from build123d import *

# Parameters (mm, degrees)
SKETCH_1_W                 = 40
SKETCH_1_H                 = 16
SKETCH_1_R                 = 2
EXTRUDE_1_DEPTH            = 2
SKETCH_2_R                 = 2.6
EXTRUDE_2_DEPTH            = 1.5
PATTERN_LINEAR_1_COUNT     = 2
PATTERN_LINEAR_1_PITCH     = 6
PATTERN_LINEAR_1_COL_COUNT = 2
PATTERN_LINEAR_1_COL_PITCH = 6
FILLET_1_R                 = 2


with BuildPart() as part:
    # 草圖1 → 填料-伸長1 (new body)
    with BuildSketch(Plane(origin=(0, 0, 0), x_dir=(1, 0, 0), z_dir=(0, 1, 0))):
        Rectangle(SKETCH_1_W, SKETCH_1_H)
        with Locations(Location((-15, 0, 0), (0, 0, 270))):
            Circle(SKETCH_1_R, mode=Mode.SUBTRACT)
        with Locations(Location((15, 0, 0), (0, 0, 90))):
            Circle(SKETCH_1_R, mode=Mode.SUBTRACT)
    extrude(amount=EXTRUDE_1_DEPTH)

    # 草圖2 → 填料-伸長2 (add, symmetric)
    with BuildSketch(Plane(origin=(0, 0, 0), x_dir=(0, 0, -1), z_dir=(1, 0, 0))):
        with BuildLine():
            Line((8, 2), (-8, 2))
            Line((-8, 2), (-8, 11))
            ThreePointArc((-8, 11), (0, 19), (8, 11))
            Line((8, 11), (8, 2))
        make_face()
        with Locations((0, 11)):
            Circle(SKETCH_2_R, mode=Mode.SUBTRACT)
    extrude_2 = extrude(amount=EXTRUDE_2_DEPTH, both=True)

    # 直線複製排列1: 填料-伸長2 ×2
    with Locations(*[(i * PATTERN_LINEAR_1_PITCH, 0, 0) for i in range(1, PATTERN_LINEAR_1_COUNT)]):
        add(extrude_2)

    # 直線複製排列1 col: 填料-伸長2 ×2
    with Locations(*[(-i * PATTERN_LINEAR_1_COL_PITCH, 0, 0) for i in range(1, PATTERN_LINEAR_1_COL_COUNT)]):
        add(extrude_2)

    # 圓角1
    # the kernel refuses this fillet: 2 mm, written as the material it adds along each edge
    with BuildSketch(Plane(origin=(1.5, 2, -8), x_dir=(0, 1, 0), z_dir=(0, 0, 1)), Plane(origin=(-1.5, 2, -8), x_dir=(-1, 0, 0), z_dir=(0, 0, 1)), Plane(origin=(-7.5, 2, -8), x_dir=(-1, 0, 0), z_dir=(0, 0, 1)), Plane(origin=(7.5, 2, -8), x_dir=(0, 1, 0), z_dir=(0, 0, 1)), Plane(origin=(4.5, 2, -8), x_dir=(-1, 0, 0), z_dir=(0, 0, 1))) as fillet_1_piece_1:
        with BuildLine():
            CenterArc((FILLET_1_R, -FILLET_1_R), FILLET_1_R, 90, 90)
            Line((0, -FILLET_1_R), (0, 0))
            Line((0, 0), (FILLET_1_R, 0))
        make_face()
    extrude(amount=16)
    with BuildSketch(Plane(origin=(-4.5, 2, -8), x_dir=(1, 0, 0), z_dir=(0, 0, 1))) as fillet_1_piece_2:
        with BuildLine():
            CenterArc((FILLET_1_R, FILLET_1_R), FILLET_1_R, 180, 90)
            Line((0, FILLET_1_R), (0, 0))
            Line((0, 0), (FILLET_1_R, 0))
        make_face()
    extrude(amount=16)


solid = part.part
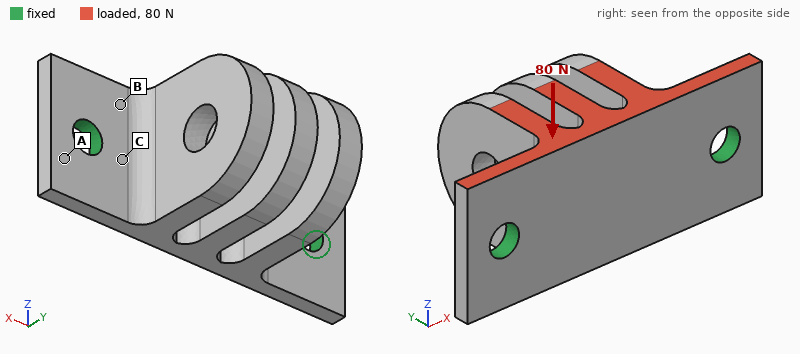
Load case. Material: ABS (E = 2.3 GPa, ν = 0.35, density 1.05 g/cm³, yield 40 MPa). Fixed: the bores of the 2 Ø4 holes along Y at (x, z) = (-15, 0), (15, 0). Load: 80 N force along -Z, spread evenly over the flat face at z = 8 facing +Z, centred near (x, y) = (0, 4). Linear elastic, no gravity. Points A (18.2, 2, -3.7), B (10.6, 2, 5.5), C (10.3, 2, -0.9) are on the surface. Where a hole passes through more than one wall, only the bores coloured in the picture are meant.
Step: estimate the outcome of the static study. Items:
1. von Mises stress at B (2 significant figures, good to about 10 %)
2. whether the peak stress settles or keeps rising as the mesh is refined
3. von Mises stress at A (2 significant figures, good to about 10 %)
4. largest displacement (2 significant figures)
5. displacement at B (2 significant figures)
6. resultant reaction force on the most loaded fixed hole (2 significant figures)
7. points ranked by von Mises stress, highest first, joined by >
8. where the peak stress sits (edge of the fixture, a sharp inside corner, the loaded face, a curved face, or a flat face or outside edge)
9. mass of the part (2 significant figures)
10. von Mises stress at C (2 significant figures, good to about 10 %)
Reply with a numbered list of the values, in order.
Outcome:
1. 4.6 MPa
2. keeps rising
3. 2.3 MPa
4. 0.28 mm
5. 0.053 mm
6. 40 N
7. C > B > A
8. edge of the fixture
9. 3.5 g
10. 7.5 MPa
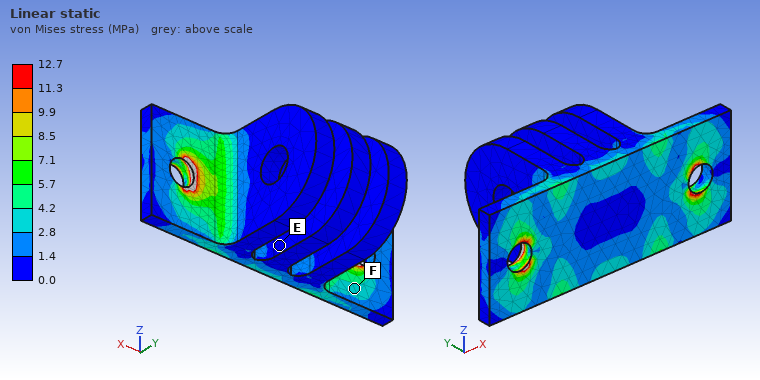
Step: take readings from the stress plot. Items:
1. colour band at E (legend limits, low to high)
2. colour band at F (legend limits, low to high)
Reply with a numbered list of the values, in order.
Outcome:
1. 0.0 to 1.4 MPa
2. 2.8 to 4.2 MPa
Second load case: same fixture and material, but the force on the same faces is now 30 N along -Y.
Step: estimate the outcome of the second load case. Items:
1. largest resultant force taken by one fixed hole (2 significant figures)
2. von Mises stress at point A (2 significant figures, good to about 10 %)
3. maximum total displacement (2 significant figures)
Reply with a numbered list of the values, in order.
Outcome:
1. 17 N
2. 2.2 MPa
3. 0.25 mm
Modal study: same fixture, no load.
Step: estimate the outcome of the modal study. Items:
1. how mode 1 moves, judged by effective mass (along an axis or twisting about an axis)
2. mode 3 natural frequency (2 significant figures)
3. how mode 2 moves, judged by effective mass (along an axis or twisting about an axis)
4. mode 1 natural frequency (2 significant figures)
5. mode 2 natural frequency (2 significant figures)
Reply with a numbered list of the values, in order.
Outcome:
1. along Z
2. 2300 Hz
3. along Y
4. 1200 Hz
5. 1500 Hz
